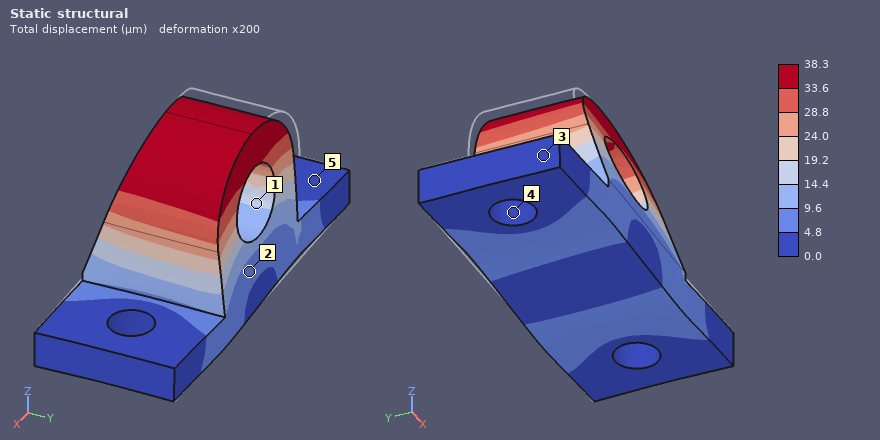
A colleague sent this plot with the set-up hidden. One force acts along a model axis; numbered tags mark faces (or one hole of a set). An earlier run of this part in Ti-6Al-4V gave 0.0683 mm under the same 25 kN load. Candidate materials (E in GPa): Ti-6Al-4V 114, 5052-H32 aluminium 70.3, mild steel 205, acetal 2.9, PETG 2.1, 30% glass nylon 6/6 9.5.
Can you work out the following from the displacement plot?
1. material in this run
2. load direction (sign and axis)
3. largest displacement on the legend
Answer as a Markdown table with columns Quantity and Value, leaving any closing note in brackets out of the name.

| Quantity | Value |
|---|---|
| material in this run | mild steel |
| load direction | +X |
| largest displacement on the legend | 38.3 µm |
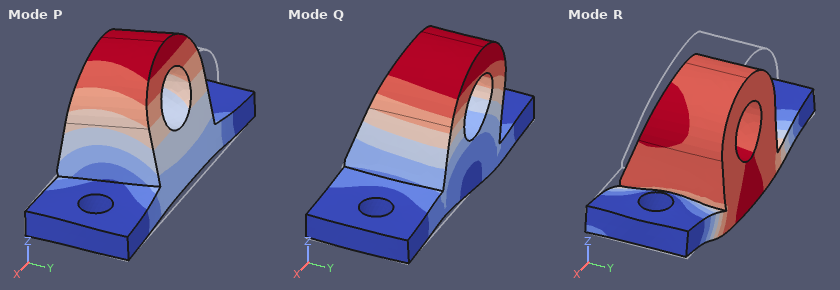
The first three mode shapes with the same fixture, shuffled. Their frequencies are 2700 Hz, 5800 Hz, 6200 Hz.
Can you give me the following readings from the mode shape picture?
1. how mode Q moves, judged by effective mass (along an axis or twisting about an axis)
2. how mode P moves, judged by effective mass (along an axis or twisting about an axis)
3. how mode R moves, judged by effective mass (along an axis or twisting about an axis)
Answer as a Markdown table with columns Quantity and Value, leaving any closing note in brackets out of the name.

| Quantity | Value |
|---|---|
| how mode Q moves, judged by effective mass | along X |
| how mode P moves, judged by effective mass | along Y |
| how mode R moves, judged by effective mass | along Z |
